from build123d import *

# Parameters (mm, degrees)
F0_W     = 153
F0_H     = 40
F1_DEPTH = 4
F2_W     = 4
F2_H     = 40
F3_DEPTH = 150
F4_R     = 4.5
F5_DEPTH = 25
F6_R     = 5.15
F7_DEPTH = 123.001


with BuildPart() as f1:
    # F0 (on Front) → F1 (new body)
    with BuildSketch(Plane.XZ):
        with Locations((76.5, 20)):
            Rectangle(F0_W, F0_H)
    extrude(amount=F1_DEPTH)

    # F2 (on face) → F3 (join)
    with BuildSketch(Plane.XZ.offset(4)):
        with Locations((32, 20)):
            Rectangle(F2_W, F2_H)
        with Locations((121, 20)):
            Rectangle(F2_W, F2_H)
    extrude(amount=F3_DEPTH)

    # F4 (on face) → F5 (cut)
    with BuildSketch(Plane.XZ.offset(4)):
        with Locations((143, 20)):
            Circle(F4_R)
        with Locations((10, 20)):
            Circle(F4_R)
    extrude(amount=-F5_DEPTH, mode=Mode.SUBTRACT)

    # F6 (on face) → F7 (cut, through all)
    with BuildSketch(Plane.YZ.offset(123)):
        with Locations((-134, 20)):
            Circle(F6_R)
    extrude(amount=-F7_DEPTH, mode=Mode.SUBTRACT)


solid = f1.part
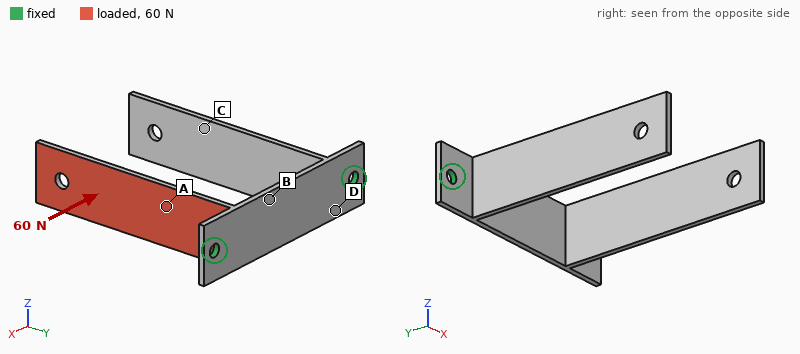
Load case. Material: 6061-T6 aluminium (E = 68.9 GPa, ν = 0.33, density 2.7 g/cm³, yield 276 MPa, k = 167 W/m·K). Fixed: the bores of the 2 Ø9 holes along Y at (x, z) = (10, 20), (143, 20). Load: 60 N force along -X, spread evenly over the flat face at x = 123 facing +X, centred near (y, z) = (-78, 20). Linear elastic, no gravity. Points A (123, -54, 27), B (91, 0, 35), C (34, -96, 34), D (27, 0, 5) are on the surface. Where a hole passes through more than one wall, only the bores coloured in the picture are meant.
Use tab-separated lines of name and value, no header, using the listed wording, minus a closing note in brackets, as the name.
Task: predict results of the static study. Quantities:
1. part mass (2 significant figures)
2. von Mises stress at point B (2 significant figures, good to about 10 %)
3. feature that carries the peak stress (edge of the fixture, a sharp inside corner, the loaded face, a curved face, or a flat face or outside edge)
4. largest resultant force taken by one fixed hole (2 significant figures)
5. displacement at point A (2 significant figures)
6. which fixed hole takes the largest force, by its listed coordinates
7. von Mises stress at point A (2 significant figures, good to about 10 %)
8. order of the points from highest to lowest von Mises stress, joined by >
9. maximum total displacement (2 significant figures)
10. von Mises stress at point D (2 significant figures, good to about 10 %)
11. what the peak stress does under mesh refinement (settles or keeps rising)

part mass	190 g
von Mises stress at point B	10 MPa
feature that carries the peak stress	edge of the fixture
largest resultant force taken by one fixed hole	59 N
displacement at point A	0.45 mm
which fixed hole takes the largest force, by its listed coordinates	(143, 20)
von Mises stress at point A	18 MPa
order of the points from highest to lowest von Mises stress, joined by >	A > B > D > C
maximum total displacement	2.1 mm
von Mises stress at point D	6.0 MPa
what the peak stress does under mesh refinement	keeps rising
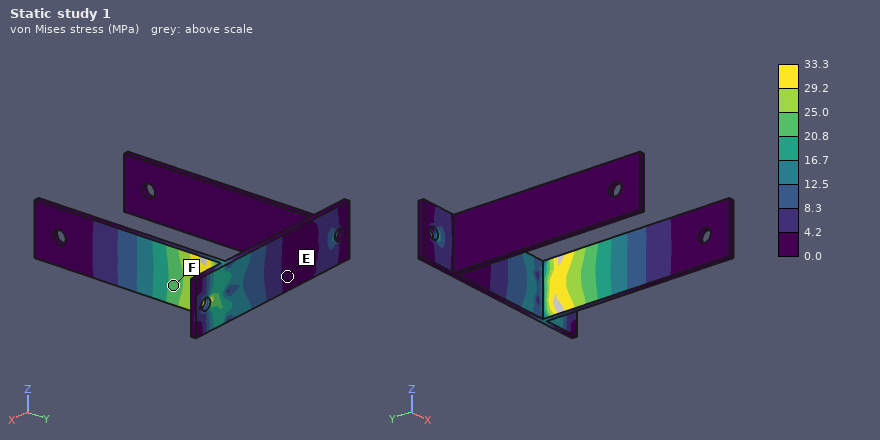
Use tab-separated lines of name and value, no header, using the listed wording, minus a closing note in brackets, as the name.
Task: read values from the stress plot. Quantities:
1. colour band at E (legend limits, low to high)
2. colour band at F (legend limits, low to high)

colour band at E	0.0 to 4.2 MPa
colour band at F	20.8 to 25.0 MPa
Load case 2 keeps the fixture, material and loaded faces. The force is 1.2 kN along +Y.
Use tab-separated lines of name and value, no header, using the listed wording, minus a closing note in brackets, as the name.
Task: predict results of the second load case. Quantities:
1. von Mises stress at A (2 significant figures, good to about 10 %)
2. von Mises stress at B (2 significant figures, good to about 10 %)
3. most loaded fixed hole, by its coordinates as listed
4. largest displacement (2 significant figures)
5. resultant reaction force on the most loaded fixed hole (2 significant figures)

von Mises stress at A	20 MPa
von Mises stress at B	24 MPa
most loaded fixed hole, by its coordinates as listed	(143, 20)
largest displacement	0.44 mm
resultant reaction force on the most loaded fixed hole	1.1 kN
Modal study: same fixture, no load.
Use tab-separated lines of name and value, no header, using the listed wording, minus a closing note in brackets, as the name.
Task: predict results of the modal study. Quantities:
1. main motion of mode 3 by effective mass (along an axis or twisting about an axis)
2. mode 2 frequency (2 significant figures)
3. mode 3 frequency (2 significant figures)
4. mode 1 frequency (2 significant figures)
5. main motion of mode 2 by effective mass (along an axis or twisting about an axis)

main motion of mode 3 by effective mass	along Z
mode 2 frequency	140 Hz
mode 3 frequency	280 Hz
mode 1 frequency	130 Hz
main motion of mode 2 by effective mass	along X
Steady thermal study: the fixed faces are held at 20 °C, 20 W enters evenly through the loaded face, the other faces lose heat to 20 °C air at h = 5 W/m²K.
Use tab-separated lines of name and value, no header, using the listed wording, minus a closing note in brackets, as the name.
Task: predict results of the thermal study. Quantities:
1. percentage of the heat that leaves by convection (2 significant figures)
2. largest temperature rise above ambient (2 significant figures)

percentage of the heat that leaves by convection	11 %
largest temperature rise above ambient	63 K
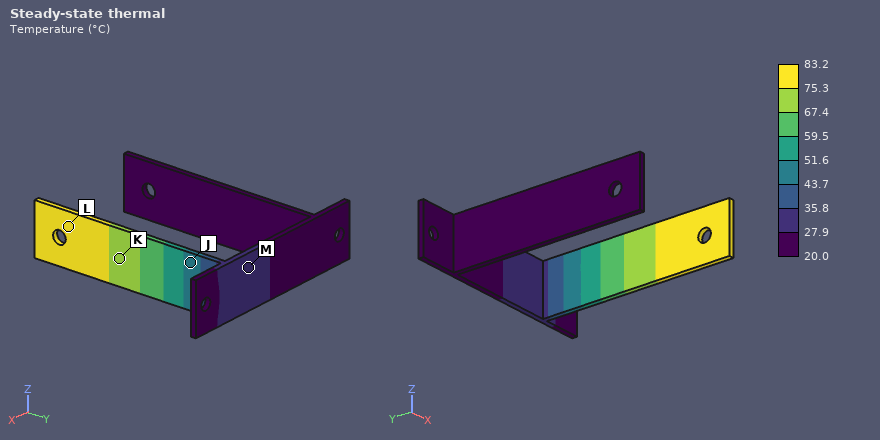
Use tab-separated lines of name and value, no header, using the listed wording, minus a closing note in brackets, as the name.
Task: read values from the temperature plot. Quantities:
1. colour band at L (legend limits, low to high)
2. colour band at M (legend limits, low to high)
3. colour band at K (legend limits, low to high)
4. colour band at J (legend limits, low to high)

colour band at L	75.3 to 83.2 °C
colour band at M	27.9 to 35.8 °C
colour band at K	67.4 to 75.3 °C
colour band at J	43.7 to 51.6 °C
